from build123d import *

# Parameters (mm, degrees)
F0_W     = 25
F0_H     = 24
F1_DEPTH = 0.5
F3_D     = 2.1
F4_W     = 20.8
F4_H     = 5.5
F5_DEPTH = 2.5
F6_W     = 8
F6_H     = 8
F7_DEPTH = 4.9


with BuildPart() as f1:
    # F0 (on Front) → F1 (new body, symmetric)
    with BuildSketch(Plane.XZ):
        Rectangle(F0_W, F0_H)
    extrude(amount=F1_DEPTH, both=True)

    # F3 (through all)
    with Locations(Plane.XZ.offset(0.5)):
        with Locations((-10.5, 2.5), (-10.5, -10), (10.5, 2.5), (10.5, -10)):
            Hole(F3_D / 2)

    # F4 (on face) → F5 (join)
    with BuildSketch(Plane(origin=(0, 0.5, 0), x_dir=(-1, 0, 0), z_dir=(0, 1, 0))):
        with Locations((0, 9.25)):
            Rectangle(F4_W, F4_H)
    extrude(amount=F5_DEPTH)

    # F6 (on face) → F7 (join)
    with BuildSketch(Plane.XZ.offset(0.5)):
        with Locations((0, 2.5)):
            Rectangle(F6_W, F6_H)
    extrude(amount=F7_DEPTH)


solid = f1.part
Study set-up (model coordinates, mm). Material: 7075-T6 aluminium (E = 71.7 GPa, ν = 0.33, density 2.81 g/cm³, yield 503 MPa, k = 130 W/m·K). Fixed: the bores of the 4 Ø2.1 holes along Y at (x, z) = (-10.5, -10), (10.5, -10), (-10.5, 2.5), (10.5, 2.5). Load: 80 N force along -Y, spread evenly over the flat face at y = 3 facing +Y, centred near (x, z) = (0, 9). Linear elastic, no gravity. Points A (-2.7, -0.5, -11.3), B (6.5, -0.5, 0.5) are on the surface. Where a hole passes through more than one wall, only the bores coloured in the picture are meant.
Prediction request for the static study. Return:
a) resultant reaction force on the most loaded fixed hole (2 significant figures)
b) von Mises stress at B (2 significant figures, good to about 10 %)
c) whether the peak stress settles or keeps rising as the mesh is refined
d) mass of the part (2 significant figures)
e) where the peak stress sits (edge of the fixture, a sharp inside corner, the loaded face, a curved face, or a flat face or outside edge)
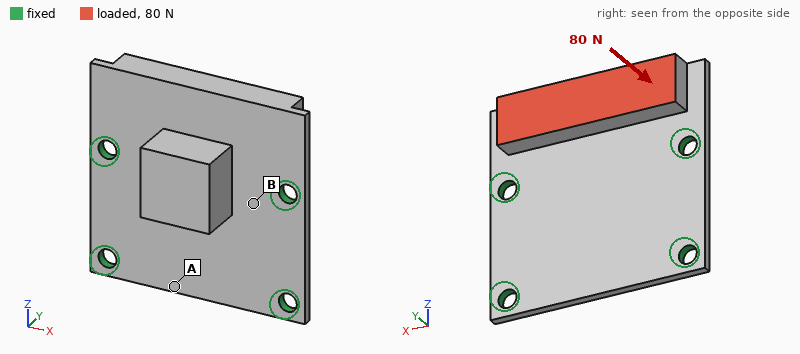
49 N
28 MPa
keeps rising
3.3 g
edge of the fixture
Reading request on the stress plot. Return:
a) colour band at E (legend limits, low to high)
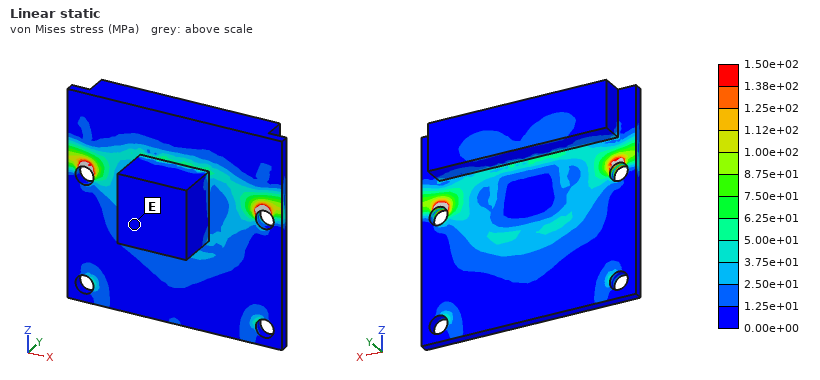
0.00e+00 to 1.25e+01 MPa
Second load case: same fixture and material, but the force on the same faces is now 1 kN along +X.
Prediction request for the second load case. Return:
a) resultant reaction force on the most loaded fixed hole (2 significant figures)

560 N
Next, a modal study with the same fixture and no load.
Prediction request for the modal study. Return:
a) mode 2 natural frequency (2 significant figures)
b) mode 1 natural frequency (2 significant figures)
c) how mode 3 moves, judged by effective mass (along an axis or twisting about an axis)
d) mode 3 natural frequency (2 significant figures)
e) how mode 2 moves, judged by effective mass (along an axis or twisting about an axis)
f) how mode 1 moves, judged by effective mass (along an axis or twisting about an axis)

11 kHz
5700 Hz
twisting about Z
17 kHz
along Y
along Y
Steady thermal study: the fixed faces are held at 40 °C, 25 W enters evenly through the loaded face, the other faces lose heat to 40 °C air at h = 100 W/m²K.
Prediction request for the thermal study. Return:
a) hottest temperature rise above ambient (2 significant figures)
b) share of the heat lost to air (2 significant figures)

54 K
13 %
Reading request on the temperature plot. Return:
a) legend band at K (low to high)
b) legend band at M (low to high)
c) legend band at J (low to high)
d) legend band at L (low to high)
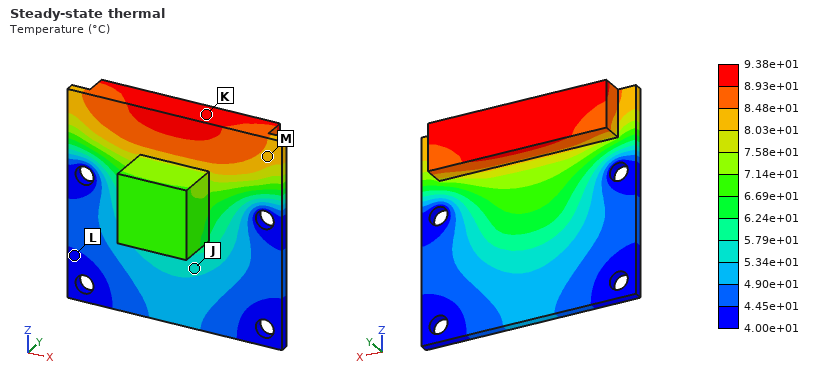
8.93e+01 to 9.38e+01 °C
8.03e+01 to 8.48e+01 °C
5.34e+01 to 5.79e+01 °C
4.00e+01 to 4.45e+01 °C
